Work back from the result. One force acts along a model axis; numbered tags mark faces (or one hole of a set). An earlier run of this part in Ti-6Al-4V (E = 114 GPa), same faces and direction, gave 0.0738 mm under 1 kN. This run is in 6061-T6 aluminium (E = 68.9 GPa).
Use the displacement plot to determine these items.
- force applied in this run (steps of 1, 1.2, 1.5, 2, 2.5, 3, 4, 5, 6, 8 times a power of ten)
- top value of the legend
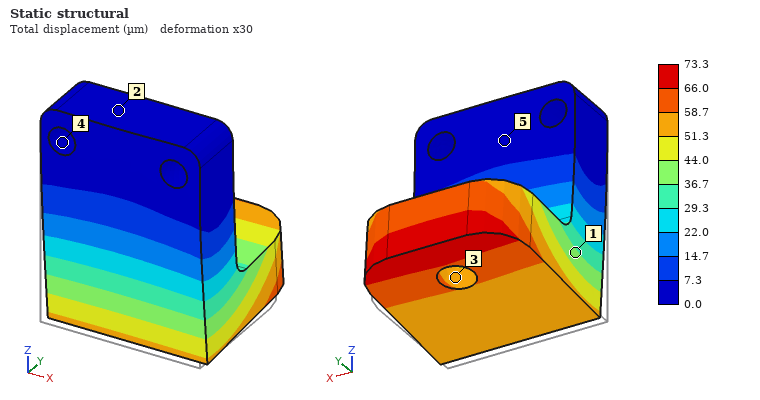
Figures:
600 N
73.3 µm
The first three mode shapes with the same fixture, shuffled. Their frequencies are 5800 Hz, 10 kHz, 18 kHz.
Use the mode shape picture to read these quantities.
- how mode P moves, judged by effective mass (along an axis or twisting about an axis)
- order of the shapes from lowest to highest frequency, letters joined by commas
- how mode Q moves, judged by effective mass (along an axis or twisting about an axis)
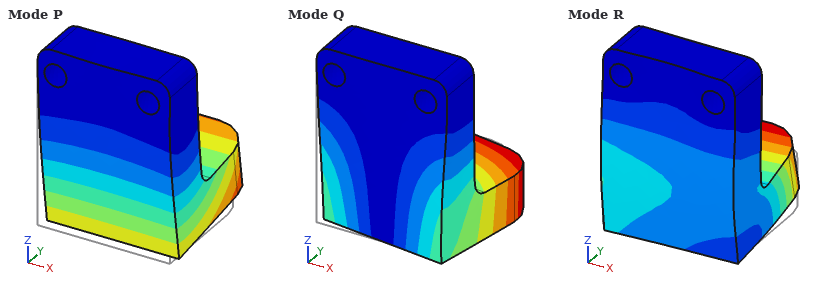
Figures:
along Y
P, Q, R
along X
